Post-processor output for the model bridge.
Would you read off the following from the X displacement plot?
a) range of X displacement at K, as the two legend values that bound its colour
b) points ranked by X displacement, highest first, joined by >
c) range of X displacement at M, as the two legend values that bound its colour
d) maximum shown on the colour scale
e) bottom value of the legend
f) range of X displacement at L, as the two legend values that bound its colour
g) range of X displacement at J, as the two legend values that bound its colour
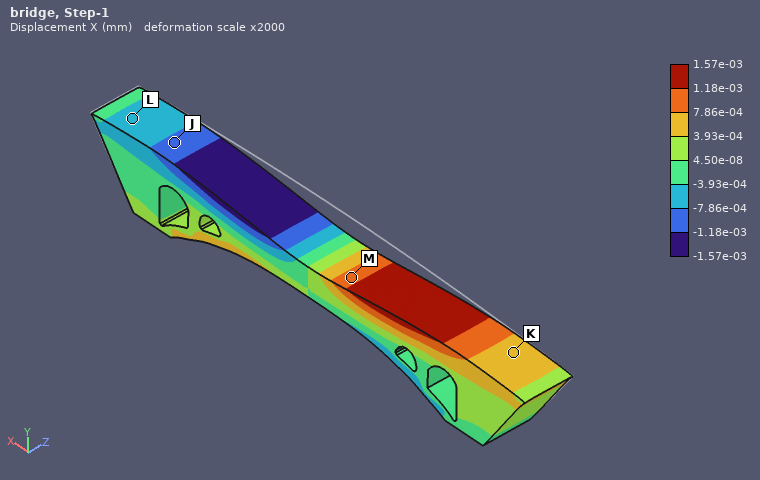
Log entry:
3.93e-04 to 7.86e-04 mm
M > K > L > J
7.86e-04 to 1.18e-03 mm
1.57e-03 mm
-1.57e-03 mm
-7.86e-04 to -3.93e-04 mm
-1.18e-03 to -7.86e-04 mm
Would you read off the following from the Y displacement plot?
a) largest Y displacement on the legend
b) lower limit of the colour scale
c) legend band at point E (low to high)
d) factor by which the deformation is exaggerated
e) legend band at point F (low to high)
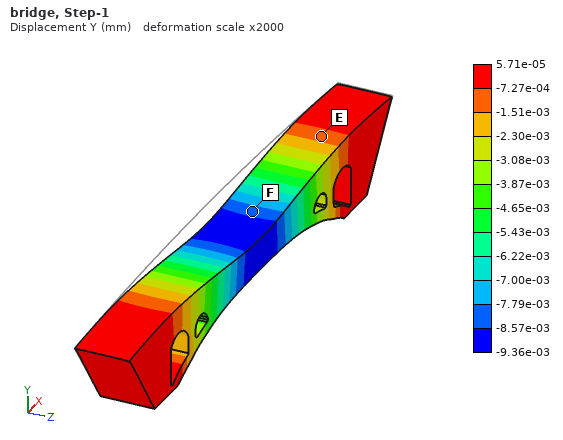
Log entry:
5.71e-05 mm
-9.36e-03 mm
-1.51e-03 to -7.27e-04 mm
2000
-8.57e-03 to -7.79e-03 mm
